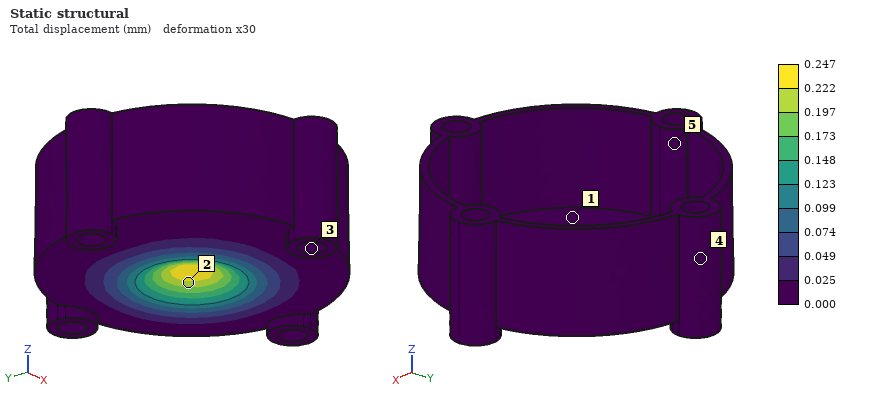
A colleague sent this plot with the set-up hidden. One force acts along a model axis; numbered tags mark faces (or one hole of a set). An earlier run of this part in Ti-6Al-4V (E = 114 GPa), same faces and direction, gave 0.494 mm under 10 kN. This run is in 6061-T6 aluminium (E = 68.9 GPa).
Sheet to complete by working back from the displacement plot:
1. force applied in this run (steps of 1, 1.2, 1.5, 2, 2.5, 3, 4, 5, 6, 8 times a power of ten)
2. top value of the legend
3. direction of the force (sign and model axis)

3 kN
0.247 mm
+Z
